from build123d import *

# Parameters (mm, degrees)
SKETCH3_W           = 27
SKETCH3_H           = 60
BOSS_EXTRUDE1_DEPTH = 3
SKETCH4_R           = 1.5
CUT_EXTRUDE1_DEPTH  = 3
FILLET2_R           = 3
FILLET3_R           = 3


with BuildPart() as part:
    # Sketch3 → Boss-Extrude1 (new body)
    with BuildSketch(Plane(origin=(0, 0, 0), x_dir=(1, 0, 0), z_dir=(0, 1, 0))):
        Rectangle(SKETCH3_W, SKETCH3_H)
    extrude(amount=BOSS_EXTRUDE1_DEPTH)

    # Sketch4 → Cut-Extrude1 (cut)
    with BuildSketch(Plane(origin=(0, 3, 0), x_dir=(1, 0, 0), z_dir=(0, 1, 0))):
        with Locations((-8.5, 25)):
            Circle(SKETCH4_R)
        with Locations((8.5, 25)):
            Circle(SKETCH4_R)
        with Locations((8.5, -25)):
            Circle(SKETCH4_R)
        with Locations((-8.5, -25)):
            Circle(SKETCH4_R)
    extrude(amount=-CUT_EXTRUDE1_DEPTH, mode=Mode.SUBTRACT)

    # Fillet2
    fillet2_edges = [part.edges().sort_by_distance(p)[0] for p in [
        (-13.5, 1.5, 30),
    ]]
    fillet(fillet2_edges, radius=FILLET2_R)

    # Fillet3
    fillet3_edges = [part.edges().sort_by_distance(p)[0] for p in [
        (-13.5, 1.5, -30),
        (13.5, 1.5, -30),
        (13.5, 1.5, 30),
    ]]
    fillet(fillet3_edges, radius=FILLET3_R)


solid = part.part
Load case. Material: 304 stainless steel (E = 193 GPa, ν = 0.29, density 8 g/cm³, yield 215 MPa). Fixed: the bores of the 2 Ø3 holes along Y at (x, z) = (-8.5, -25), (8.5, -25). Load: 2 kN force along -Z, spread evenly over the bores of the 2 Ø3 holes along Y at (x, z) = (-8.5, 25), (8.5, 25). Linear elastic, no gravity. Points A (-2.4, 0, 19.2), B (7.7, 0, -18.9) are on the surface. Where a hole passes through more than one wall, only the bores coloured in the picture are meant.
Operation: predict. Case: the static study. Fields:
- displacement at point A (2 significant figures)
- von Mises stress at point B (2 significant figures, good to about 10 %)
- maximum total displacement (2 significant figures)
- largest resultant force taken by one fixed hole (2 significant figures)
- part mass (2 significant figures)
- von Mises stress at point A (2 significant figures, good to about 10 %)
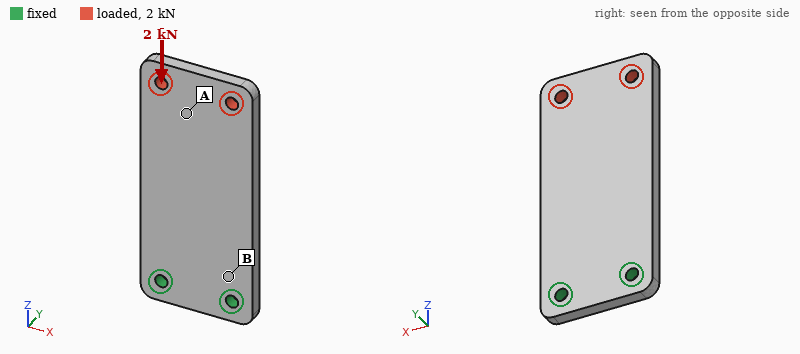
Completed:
5.8 µm
32 MPa
7.8 µm
1.0 kN
38 g
19 MPa
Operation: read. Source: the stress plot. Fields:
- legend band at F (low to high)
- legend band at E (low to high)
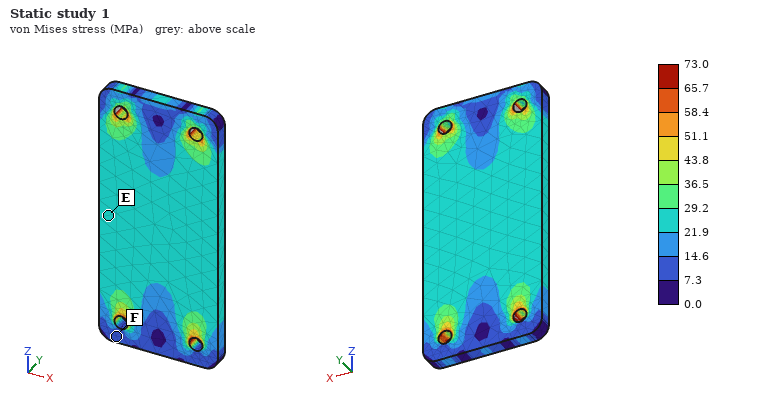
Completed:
7.3 to 14.6 MPa
21.9 to 29.2 MPa
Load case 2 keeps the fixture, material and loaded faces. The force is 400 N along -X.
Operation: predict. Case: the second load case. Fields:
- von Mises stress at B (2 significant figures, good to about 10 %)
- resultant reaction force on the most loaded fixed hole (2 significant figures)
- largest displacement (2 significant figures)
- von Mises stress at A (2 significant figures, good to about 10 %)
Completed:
36 MPa
1.1 kN
27 µm
12 MPa
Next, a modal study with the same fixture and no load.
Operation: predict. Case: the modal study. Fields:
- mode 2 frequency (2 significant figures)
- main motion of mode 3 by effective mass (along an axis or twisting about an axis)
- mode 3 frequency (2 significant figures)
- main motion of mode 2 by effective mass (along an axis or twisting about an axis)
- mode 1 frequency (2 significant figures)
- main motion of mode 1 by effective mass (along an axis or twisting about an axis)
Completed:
3500 Hz
along Y
4900 Hz
twisting about Z
810 Hz
along Y
